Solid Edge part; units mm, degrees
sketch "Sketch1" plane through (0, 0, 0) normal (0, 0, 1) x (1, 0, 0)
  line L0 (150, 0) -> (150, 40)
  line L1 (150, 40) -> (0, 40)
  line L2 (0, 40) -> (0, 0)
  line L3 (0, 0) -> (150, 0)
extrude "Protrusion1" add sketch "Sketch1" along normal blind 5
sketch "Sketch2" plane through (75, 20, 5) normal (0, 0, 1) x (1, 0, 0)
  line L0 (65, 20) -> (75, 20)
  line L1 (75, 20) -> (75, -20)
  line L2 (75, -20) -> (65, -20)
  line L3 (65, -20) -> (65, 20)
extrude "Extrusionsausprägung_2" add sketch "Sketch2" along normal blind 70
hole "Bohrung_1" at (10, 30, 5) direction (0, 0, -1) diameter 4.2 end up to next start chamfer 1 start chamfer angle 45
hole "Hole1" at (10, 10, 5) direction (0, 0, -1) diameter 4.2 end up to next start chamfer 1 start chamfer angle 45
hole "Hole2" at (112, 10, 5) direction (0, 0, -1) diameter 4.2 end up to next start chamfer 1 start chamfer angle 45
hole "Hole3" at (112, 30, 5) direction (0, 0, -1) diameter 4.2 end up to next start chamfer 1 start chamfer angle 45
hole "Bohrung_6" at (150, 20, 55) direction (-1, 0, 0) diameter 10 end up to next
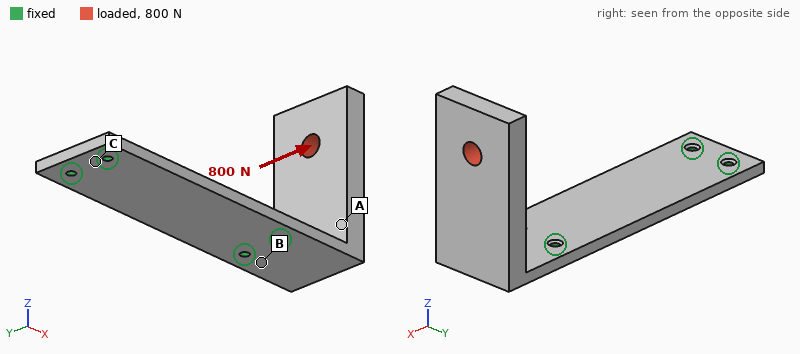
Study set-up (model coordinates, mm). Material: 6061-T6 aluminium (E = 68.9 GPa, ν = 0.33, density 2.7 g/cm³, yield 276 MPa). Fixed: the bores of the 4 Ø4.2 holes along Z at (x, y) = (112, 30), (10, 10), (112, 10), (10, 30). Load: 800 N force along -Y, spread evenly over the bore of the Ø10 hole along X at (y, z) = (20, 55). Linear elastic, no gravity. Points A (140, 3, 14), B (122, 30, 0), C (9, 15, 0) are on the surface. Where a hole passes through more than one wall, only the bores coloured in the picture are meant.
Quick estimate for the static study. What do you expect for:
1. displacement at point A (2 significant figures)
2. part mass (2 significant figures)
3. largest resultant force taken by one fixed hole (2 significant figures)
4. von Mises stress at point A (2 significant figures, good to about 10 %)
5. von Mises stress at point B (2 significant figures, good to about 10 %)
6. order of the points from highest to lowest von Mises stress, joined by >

0.35 mm
150 g
2.0 kN
36 MPa
140 MPa
B > A > C
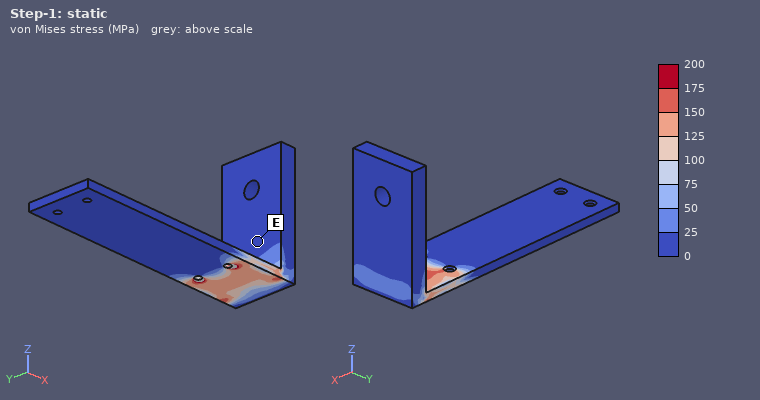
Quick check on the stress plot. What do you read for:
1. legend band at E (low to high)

0 to 25 MPa
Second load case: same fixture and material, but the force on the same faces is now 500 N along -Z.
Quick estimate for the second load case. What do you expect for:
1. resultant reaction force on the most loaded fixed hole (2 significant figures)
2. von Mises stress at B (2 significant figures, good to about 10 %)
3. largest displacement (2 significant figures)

260 N
63 MPa
0.75 mm
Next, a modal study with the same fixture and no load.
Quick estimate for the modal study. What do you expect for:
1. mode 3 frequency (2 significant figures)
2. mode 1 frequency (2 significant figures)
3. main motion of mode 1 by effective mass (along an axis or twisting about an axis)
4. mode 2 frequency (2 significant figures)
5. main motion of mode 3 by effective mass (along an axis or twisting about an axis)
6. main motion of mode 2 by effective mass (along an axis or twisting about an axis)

1800 Hz
380 Hz
along X
660 Hz
along Z
along Y
